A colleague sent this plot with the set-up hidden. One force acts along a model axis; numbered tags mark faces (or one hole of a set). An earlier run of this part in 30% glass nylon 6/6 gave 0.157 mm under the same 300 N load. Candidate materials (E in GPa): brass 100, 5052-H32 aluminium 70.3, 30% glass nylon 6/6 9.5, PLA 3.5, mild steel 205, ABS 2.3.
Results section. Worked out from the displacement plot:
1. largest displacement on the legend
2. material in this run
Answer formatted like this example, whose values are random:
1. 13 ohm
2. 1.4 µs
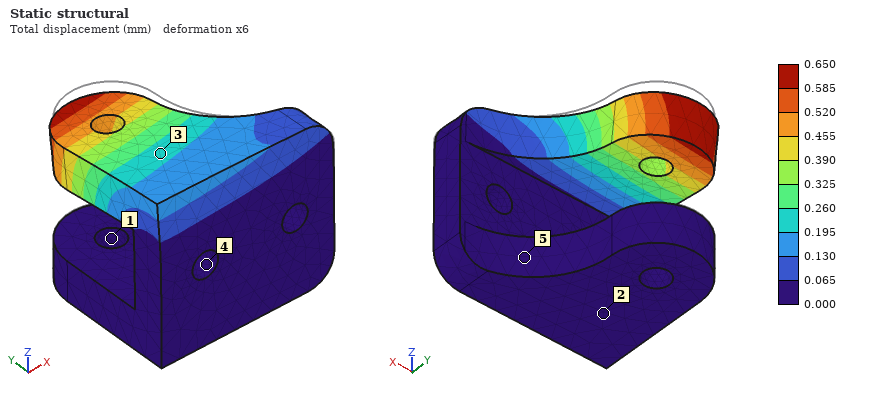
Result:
1. 0.650 mm
2. ABS
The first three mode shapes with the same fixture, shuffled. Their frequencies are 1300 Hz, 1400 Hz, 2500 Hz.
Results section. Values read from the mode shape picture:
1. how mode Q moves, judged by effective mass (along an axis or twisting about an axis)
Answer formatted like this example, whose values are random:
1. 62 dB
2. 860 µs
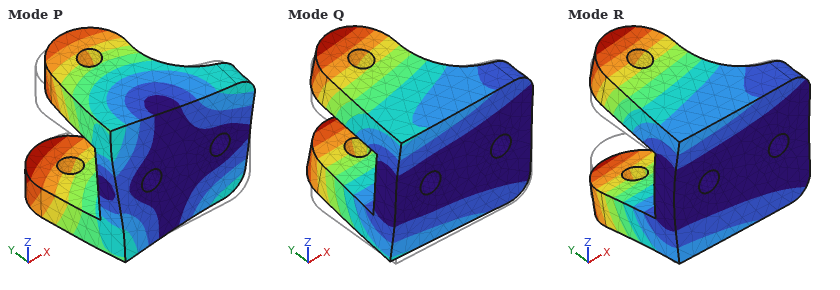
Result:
1. along Z
